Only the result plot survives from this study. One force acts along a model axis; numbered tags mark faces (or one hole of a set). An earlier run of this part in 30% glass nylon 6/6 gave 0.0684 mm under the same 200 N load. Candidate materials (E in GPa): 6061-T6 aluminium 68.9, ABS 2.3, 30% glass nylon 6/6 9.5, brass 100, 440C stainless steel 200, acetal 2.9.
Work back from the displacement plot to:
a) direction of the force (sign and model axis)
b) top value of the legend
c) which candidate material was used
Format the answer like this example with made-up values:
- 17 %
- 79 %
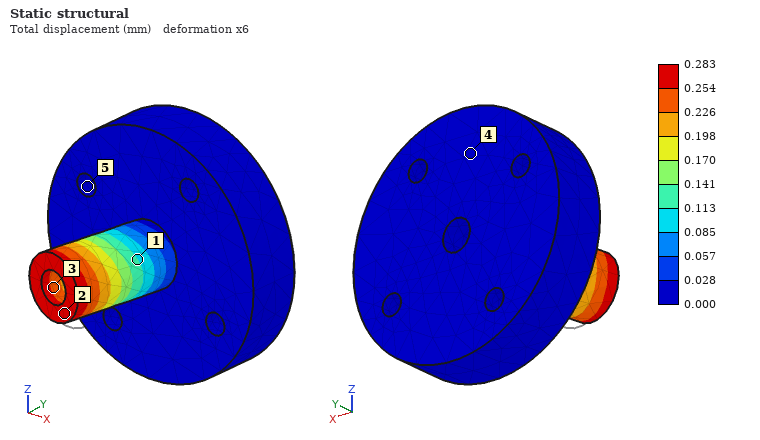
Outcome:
- -X
- 0.283 mm
- ABS
